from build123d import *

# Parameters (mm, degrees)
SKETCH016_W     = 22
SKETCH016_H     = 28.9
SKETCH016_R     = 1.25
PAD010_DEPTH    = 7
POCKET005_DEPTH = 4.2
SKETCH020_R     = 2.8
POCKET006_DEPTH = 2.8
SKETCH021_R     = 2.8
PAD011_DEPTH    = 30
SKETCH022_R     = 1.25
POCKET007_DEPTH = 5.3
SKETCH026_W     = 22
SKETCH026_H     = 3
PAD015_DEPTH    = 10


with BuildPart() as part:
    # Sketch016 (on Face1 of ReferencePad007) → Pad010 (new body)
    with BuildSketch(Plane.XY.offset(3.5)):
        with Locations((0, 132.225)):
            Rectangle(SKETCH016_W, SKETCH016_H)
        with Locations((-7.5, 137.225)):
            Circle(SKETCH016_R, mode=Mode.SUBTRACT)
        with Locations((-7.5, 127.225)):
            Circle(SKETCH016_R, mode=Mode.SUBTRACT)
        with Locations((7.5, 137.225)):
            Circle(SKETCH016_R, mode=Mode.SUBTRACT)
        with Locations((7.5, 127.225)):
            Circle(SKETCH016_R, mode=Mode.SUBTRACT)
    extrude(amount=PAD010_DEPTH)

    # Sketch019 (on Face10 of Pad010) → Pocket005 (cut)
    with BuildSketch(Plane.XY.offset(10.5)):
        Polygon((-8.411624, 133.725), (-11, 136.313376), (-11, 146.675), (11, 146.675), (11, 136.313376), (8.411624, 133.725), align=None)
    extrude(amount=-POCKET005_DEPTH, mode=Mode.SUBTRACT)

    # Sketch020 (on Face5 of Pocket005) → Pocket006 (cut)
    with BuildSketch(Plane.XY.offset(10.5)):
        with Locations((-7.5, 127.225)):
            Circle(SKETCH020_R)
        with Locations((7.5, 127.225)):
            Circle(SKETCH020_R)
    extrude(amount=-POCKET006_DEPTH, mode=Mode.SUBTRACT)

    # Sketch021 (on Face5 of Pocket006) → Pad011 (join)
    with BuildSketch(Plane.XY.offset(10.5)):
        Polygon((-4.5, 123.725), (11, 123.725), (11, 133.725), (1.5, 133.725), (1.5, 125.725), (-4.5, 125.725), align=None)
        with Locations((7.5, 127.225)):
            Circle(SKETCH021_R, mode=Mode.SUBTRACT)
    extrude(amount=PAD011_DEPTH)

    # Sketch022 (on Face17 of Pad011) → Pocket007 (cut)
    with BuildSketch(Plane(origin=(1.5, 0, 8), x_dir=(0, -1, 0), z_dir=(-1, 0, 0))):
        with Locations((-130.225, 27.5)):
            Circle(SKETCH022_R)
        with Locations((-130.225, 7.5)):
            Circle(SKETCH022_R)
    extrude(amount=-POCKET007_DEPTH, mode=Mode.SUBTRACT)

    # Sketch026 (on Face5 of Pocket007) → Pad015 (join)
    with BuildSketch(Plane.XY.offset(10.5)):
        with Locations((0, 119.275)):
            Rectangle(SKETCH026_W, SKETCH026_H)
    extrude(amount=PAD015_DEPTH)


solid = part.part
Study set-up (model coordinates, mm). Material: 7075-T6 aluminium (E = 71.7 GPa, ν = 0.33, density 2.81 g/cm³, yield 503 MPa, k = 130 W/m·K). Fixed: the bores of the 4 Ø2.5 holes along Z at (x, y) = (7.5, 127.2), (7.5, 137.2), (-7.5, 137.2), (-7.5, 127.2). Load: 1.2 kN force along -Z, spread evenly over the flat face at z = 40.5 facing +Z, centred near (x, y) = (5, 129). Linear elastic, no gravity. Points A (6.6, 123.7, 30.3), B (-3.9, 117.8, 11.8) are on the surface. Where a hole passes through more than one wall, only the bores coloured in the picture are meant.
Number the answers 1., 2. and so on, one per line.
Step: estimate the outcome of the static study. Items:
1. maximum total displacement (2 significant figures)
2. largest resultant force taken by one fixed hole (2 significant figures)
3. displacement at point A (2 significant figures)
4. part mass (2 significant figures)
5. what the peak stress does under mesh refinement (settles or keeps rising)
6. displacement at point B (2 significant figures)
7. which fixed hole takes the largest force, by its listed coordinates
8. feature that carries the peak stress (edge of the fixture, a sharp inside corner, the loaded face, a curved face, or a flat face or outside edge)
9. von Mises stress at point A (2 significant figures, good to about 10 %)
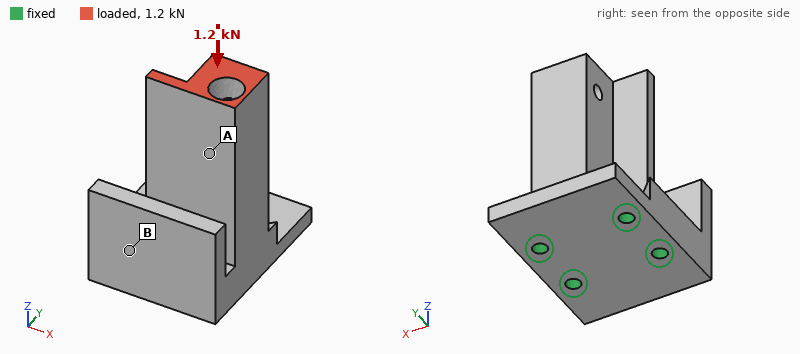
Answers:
1. 9.8 µm
2. 760 N
3. 6.2 µm
4. 17 g
5. keeps rising
6. 1.7 µm
7. (7.5, 127.2)
8. edge of the fixture
9. 15 MPa
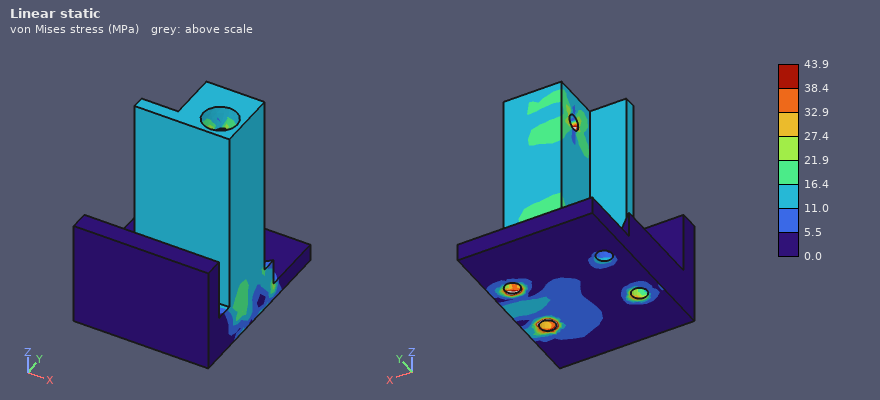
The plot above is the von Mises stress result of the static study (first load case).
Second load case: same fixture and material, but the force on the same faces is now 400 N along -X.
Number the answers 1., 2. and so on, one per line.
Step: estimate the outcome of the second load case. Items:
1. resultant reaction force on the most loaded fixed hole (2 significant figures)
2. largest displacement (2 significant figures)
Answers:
1. 800 N
2. 98 µm
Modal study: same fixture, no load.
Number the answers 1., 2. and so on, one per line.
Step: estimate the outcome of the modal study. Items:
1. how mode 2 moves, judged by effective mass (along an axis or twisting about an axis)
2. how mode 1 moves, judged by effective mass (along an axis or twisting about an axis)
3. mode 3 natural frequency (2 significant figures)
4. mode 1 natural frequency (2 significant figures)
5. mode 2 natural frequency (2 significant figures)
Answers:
1. along X
2. along Y
3. 14 kHz
4. 5500 Hz
5. 7900 Hz
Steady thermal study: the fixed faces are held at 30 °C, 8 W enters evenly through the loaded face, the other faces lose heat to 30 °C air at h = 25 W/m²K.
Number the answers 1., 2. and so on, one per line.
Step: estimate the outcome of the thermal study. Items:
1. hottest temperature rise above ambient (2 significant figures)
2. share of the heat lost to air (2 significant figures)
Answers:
1. 25 K
2. 9.9 %
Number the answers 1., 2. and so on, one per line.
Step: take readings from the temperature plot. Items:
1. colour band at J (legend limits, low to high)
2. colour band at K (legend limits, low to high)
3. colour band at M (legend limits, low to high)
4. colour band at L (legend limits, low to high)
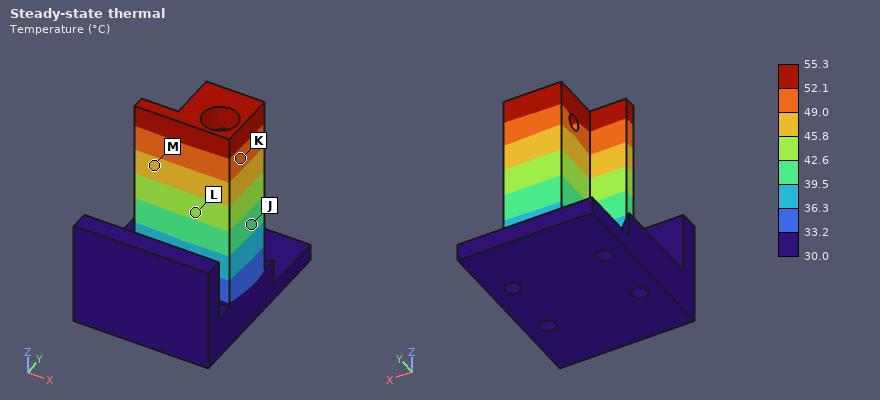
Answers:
1. 39.5 to 42.6 °C
2. 49.0 to 52.1 °C
3. 45.8 to 49.0 °C
4. 42.6 to 45.8 °C
